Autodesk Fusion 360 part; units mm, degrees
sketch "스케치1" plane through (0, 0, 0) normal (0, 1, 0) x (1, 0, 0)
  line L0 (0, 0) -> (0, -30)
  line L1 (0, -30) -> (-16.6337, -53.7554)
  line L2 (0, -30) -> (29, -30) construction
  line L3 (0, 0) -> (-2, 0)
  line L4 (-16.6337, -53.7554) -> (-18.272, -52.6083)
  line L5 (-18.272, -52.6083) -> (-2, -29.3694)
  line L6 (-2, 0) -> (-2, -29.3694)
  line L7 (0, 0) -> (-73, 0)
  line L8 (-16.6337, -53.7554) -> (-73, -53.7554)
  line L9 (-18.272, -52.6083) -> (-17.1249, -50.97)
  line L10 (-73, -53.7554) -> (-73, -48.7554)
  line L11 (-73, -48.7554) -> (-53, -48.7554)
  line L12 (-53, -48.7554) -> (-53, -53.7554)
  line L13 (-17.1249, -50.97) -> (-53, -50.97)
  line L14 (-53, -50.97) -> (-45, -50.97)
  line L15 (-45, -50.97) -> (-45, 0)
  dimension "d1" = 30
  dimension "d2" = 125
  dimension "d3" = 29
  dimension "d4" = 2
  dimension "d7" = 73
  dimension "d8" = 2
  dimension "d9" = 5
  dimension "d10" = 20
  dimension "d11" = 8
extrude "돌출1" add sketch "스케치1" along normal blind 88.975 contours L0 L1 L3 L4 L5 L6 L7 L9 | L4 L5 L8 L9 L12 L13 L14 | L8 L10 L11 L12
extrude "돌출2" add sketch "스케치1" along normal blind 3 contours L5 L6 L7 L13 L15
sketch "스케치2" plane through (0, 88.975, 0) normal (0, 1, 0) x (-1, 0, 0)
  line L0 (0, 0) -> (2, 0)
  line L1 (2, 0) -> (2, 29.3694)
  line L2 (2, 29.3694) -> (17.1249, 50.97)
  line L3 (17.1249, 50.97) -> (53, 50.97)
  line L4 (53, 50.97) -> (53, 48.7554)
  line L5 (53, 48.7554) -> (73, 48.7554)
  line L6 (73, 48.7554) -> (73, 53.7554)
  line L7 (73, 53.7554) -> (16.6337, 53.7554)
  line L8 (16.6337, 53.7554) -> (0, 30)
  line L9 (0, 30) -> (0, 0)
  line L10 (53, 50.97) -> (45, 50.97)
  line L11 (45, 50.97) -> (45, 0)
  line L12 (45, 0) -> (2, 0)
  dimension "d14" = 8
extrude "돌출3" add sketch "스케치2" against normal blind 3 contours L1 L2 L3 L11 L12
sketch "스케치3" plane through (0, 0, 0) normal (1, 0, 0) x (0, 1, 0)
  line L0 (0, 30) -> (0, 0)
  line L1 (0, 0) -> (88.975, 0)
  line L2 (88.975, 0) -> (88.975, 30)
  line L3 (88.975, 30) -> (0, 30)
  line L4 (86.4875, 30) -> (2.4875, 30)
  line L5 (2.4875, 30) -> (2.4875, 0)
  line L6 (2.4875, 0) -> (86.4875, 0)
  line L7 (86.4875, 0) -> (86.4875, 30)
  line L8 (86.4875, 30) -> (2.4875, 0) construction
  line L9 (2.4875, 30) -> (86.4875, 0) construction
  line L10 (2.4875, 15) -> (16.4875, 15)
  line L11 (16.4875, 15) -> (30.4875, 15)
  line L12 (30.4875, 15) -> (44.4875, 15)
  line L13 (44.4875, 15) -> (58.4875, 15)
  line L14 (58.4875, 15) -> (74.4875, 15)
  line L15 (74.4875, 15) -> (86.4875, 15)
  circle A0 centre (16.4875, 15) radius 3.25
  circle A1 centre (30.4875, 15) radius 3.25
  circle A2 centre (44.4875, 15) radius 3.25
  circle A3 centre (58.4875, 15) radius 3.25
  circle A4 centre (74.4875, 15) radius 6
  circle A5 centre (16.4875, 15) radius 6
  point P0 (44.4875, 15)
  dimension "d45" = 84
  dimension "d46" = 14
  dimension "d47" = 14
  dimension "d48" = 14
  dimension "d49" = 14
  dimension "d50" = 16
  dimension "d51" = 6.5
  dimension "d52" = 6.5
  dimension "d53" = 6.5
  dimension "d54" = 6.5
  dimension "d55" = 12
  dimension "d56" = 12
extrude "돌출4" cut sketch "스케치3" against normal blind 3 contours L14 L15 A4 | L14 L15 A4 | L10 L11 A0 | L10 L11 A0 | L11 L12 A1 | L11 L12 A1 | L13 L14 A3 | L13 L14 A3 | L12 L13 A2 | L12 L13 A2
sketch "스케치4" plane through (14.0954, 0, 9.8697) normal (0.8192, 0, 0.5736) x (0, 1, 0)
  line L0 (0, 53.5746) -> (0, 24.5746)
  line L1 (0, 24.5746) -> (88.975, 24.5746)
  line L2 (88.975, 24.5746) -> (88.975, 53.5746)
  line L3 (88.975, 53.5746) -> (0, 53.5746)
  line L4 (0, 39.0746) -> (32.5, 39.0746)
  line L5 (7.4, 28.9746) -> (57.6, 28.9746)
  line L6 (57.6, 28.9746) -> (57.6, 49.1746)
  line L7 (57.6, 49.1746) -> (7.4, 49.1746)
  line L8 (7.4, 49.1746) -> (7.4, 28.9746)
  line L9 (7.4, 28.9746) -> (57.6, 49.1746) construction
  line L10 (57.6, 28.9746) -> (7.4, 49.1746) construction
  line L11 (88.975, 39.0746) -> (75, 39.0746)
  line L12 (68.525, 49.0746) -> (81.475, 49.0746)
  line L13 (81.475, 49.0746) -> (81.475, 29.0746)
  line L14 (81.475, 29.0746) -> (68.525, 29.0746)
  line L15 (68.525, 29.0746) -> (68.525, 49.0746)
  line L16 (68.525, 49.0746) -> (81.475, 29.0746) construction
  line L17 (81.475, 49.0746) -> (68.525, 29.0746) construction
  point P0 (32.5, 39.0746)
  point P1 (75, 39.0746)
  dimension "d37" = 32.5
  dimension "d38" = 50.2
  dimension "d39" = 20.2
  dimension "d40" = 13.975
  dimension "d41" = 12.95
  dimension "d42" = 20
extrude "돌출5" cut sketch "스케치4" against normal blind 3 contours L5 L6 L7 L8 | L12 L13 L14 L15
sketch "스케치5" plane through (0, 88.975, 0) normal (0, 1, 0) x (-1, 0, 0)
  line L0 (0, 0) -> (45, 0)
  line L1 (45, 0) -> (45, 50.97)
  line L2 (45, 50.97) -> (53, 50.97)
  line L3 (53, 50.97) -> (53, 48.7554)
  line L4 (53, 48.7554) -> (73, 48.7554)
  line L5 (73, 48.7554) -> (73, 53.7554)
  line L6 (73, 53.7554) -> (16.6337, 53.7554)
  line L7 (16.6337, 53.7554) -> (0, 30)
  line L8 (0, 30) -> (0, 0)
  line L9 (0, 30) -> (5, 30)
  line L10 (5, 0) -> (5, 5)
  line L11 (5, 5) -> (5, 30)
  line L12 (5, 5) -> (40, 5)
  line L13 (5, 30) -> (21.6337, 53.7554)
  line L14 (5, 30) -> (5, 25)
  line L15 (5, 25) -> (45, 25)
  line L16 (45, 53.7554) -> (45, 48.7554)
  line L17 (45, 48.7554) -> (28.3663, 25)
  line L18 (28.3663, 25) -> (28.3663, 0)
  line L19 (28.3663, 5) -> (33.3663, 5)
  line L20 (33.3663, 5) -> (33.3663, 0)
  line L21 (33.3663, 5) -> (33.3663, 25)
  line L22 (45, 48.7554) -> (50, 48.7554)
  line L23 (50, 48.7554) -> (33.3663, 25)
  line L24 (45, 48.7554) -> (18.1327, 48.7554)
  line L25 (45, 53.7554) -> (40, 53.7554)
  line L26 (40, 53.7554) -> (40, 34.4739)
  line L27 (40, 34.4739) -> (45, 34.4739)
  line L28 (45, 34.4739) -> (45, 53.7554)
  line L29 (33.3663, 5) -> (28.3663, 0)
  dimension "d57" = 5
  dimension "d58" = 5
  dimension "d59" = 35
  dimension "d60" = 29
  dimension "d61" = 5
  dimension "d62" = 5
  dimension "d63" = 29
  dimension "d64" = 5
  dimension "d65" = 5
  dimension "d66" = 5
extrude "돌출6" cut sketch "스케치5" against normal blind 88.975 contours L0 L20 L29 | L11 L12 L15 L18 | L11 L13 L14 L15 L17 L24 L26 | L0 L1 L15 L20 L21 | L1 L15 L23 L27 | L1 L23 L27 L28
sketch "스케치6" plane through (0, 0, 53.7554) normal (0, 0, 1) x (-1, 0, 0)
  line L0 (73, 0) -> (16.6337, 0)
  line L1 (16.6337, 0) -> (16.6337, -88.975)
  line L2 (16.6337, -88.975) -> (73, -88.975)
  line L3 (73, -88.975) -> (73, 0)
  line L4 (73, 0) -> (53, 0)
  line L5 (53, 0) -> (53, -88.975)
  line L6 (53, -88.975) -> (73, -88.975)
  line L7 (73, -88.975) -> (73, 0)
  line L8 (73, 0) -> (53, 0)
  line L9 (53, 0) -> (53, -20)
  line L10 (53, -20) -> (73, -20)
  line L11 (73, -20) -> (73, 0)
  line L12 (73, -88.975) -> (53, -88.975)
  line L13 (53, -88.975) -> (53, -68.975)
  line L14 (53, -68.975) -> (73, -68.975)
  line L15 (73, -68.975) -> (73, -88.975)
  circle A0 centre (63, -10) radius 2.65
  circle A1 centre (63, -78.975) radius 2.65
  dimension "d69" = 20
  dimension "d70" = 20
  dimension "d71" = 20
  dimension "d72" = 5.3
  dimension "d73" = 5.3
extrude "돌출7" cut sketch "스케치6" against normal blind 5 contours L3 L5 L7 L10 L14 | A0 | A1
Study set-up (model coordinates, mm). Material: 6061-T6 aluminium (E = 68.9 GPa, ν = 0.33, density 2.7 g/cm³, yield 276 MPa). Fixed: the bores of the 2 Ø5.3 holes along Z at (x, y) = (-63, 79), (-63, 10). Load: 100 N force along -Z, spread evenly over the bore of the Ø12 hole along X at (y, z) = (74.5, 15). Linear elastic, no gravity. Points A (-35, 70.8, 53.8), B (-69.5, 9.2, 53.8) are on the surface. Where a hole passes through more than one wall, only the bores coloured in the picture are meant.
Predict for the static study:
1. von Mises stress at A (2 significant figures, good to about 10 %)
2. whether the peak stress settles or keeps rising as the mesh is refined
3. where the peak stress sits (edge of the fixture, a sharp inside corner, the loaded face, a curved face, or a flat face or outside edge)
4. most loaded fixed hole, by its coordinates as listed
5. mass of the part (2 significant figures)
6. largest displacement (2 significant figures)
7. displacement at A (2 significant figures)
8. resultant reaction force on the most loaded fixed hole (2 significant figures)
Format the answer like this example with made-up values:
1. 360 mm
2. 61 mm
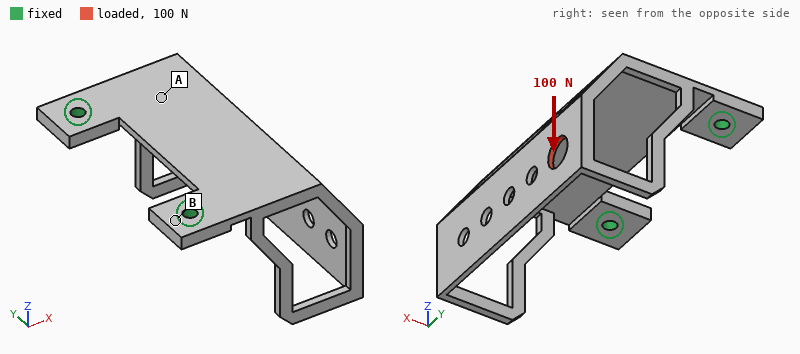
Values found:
1. 29 MPa
2. keeps rising
3. a sharp inside corner
4. (-63, 79)
5. 63 g
6. 1.3 mm
7. 0.20 mm
8. 90 N
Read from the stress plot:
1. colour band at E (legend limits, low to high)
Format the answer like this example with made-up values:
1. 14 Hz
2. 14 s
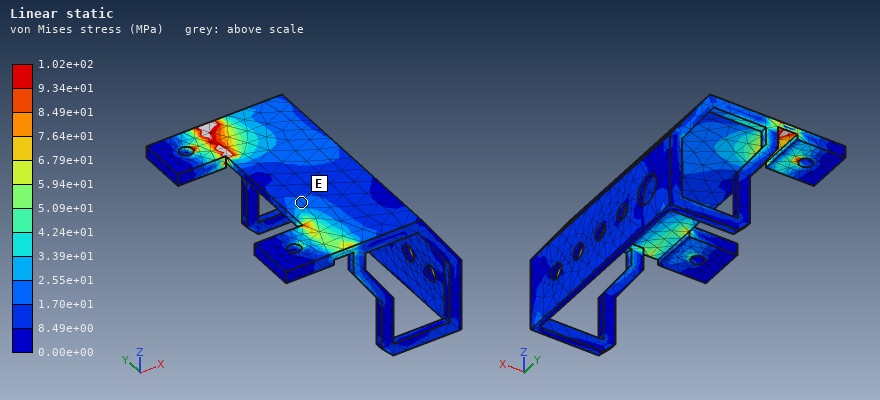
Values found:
1. 1.70e+01 to 2.55e+01 MPa
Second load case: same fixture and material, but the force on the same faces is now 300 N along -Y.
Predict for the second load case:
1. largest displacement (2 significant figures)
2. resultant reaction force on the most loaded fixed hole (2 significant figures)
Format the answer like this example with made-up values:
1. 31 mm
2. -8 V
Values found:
1. 1.2 mm
2. 320 N
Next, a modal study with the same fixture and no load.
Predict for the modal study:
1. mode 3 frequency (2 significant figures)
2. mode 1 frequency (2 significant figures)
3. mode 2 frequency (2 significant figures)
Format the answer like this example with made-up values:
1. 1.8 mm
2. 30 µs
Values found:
1. 1200 Hz
2. 320 Hz
3. 510 Hz
